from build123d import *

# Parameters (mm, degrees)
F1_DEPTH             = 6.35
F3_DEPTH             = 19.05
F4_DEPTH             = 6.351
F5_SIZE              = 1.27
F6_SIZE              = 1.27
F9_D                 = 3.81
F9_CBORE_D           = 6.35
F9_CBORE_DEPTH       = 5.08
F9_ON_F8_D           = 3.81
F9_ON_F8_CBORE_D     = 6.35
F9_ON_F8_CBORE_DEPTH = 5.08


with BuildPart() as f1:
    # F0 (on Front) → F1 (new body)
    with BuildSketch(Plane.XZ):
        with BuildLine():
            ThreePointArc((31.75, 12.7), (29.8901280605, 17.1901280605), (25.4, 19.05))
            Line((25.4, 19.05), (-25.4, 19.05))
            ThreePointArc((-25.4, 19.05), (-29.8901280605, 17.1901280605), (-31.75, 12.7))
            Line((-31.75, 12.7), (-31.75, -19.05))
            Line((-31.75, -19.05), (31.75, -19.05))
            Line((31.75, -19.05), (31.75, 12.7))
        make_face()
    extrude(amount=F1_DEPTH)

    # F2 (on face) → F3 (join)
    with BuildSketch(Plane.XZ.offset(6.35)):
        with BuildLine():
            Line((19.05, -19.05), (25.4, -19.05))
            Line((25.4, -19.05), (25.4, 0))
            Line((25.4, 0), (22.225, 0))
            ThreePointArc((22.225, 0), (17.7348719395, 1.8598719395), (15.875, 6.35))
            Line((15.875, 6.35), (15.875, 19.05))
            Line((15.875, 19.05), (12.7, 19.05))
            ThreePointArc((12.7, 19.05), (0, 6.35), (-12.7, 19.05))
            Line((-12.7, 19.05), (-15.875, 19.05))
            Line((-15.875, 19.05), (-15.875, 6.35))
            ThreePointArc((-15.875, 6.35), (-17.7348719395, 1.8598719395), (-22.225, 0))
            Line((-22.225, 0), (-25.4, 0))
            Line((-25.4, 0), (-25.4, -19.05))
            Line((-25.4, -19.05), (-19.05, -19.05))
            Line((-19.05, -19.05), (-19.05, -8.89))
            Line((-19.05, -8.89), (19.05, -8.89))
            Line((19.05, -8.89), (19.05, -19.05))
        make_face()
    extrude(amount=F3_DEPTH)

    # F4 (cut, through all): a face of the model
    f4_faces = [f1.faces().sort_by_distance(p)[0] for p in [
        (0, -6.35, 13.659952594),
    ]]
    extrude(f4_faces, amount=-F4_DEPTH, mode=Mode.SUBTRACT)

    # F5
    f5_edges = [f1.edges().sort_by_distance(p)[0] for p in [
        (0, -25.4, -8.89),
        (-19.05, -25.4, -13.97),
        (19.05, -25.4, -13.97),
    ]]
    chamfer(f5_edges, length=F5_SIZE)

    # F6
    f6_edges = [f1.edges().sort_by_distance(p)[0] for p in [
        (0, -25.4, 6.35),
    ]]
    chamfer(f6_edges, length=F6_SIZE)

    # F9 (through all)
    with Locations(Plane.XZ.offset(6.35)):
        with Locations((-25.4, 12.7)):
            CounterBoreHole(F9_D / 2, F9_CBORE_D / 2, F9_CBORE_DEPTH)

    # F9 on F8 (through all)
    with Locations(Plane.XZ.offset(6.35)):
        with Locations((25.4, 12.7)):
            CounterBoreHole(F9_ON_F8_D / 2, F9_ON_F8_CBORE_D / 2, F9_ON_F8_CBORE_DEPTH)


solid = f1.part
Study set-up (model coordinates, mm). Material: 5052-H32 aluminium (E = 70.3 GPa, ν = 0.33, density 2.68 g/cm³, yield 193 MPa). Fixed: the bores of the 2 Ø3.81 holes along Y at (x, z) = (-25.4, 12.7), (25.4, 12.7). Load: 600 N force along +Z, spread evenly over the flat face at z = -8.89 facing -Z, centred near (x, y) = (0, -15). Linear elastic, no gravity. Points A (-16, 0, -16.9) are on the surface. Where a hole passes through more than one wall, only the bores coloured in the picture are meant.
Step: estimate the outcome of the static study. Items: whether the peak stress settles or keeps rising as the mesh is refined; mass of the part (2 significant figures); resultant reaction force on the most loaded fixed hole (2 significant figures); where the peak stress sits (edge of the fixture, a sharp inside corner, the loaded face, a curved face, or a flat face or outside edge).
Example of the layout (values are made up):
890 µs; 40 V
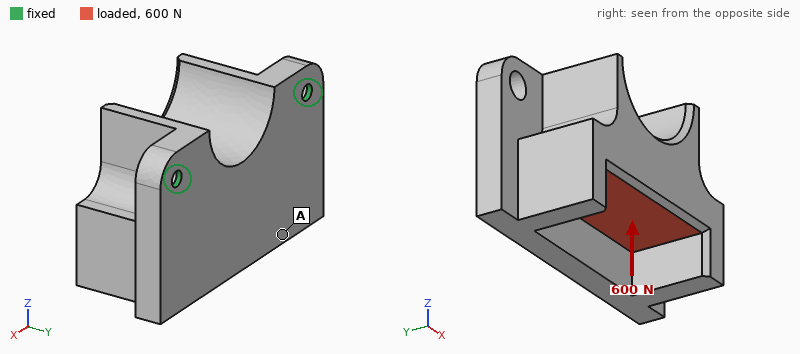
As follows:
keeps rising; 84 g; 360 N; edge of the fixture
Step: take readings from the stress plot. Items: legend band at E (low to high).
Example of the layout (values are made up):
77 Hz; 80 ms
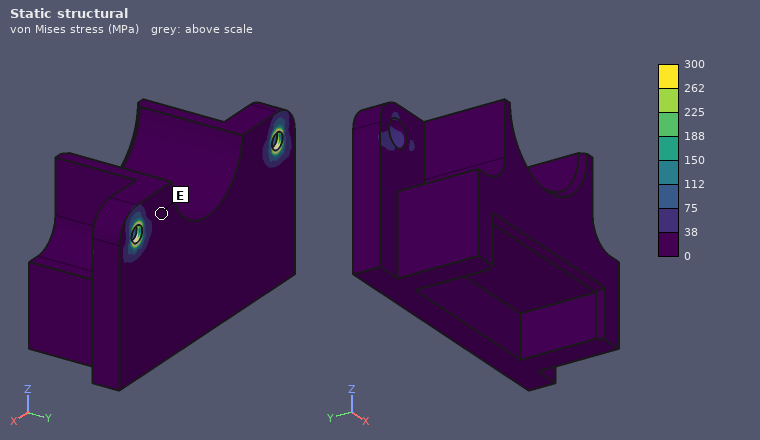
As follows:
0 to 38 MPa
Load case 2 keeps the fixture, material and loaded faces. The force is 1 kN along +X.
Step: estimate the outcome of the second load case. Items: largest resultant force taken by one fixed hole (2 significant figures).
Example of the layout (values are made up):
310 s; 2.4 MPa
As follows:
710 N
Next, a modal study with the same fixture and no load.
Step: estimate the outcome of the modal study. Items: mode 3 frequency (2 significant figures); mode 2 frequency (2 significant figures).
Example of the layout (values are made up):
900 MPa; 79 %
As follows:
7700 Hz; 6100 Hz
